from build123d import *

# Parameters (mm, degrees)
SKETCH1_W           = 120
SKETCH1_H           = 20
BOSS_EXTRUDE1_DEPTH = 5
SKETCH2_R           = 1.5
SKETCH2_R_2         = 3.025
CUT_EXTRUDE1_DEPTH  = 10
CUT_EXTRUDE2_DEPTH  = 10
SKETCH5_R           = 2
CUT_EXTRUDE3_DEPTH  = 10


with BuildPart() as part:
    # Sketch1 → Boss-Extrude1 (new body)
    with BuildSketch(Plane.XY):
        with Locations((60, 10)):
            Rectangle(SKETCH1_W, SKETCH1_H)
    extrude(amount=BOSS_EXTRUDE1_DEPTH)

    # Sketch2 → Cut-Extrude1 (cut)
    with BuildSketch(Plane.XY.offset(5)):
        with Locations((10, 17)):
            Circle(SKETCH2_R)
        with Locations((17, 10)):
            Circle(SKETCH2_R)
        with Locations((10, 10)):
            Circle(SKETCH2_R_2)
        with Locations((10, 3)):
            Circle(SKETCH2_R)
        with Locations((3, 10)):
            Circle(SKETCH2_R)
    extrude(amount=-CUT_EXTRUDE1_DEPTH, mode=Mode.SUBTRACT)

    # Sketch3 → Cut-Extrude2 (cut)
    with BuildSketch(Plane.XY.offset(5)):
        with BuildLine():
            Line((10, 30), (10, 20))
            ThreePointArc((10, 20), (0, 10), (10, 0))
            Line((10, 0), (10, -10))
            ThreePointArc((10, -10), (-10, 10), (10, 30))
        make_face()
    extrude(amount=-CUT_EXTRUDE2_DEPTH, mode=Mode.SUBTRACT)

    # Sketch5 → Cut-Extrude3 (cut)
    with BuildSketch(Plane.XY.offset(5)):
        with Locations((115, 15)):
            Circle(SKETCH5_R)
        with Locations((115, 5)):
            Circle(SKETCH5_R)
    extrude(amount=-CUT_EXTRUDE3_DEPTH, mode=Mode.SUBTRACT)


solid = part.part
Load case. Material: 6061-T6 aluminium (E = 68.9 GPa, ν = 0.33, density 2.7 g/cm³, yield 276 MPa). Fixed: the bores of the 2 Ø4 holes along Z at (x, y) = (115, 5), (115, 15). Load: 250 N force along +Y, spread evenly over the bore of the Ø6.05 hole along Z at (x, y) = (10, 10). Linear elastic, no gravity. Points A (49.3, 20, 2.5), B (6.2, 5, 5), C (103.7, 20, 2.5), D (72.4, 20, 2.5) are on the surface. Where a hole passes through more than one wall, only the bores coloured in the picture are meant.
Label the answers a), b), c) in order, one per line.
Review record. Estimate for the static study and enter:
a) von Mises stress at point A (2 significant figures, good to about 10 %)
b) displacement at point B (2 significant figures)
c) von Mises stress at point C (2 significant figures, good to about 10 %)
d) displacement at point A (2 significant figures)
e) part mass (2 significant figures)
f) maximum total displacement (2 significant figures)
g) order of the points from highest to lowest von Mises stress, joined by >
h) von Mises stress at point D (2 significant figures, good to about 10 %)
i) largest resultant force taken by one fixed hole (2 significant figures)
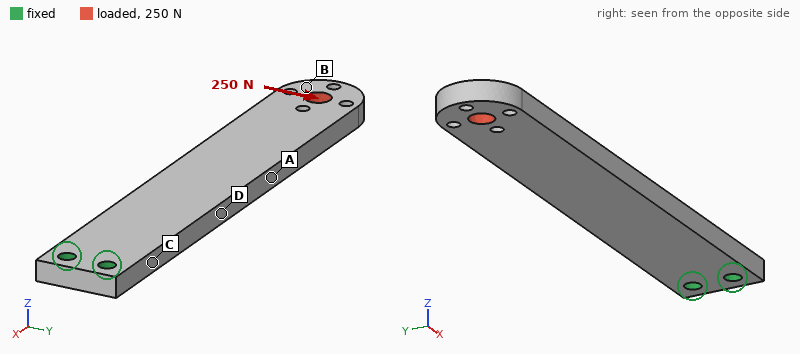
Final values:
a) 29 MPa
b) 0.46 mm
c) 69 MPa
d) 0.21 mm
e) 31 g
f) 0.50 mm
g) C > D > A > B
h) 47 MPa
i) 2.1 kN
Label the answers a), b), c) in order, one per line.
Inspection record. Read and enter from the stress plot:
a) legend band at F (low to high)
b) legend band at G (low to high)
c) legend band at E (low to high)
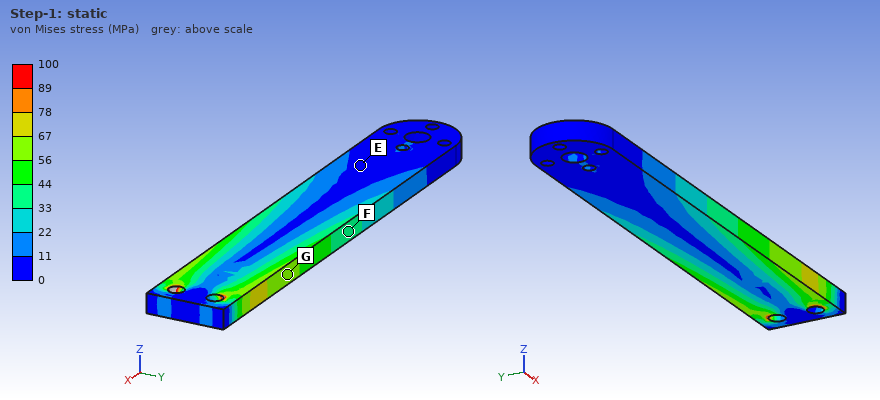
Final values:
a) 33 to 44 MPa
b) 56 to 67 MPa
c) 0 to 11 MPa
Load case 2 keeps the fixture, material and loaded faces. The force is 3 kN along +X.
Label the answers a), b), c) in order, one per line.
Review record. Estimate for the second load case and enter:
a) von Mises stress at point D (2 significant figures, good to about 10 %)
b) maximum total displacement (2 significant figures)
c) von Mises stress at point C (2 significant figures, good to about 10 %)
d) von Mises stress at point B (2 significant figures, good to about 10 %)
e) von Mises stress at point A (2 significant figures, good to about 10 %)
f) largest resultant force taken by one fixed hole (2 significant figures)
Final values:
a) 30 MPa
b) 52 µm
c) 28 MPa
d) 13 MPa
e) 30 MPa
f) 1.5 kN
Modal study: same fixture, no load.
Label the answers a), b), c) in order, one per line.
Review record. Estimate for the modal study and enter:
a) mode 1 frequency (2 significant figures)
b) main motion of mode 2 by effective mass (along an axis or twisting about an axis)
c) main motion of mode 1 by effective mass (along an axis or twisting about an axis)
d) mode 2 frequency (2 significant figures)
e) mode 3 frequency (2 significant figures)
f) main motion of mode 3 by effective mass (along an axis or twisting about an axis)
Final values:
a) 340 Hz
b) along Y
c) along Z
d) 1300 Hz
e) 2100 Hz
f) along Z
